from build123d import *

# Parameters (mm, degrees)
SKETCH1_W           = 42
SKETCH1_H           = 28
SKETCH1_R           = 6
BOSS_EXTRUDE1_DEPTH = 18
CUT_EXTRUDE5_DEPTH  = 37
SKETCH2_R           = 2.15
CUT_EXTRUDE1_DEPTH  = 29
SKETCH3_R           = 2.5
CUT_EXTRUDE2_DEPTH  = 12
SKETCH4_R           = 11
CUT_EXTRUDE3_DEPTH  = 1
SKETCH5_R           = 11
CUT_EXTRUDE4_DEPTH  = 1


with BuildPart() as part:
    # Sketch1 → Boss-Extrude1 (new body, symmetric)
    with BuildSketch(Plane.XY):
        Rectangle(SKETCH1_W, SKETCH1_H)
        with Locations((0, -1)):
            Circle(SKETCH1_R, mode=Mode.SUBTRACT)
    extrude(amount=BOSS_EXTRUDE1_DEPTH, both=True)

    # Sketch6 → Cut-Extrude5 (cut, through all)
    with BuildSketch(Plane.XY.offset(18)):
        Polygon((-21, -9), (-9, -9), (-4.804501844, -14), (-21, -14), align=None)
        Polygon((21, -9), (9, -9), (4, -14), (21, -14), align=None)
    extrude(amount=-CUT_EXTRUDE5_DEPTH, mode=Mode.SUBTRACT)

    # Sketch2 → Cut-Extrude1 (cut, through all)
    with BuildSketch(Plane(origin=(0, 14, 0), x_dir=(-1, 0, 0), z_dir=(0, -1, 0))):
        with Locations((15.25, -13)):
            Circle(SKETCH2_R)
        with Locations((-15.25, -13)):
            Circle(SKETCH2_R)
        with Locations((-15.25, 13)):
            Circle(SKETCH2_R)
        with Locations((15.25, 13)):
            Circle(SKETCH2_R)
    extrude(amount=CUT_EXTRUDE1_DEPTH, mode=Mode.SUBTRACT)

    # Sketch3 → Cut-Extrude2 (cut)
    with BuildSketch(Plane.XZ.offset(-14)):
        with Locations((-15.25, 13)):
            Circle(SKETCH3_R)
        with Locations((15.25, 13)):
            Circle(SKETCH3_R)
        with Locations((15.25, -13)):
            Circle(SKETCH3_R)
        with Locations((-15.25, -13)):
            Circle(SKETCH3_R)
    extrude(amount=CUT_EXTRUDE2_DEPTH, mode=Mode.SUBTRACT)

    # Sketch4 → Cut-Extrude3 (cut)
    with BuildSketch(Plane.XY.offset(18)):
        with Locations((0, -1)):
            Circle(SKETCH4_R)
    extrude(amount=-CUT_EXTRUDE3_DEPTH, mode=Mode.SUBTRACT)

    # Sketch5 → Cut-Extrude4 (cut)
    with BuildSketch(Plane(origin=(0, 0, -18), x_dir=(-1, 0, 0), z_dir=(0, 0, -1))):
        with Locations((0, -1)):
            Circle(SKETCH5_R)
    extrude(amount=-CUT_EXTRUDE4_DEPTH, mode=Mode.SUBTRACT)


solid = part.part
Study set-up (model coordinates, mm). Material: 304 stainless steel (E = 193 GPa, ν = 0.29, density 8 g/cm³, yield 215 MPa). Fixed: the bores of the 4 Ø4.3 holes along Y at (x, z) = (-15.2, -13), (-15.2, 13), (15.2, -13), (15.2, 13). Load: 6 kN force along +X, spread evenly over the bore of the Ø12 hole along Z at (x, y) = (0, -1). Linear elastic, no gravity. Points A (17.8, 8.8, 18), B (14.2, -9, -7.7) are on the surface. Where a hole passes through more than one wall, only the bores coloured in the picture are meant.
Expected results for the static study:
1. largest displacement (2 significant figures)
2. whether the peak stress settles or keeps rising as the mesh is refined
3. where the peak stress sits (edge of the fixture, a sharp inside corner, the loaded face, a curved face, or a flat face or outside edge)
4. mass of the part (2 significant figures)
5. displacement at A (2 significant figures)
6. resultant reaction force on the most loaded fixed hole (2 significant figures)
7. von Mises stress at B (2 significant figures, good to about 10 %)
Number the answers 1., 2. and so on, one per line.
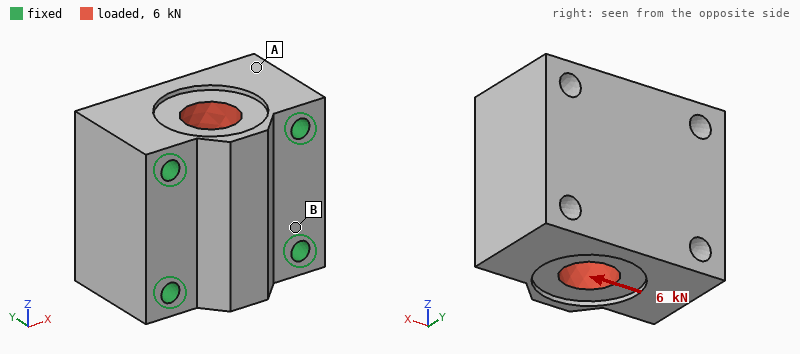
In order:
1. 0.84 µm
2. keeps rising
3. edge of the fixture
4. 250 g
5. 0.48 µm
6. 1.5 kN
7. 6.1 MPa
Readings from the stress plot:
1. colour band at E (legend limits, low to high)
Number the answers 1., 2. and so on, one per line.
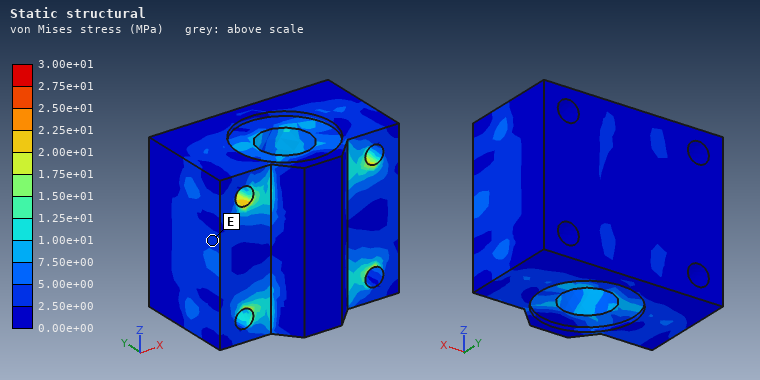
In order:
1. 2.50e+00 to 5.00e+00 MPa
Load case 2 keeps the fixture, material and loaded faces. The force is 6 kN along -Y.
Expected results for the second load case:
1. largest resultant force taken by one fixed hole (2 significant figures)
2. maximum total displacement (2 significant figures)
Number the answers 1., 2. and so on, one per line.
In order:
1. 1.5 kN
2. 1.3 µm
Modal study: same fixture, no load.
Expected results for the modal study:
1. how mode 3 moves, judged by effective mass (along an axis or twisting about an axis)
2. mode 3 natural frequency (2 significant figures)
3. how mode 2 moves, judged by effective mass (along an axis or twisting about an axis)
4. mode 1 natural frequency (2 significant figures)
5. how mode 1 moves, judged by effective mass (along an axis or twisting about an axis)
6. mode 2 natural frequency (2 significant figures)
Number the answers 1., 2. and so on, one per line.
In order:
1. along Y
2. 33 kHz
3. along Z
4. 28 kHz
5. along X
6. 29 kHz
